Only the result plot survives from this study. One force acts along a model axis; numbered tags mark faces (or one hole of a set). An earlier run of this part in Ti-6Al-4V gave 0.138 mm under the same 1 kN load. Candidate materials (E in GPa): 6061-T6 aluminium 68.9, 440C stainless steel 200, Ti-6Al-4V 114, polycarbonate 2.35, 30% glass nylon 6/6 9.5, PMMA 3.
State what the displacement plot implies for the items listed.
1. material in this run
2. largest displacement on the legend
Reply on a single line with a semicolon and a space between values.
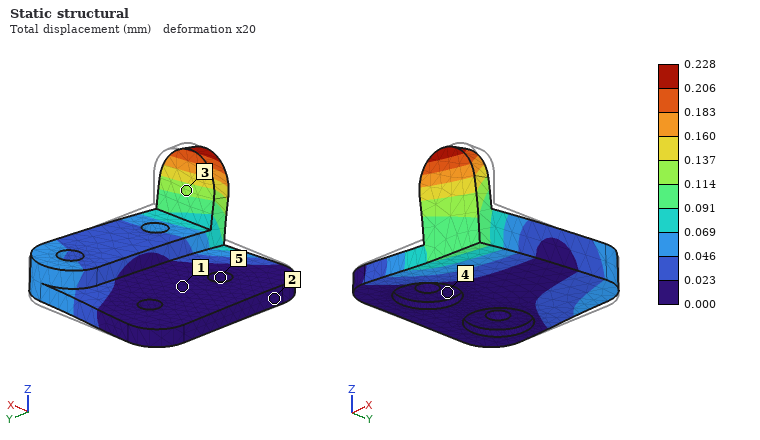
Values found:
6061-T6 aluminium; 0.228 mm
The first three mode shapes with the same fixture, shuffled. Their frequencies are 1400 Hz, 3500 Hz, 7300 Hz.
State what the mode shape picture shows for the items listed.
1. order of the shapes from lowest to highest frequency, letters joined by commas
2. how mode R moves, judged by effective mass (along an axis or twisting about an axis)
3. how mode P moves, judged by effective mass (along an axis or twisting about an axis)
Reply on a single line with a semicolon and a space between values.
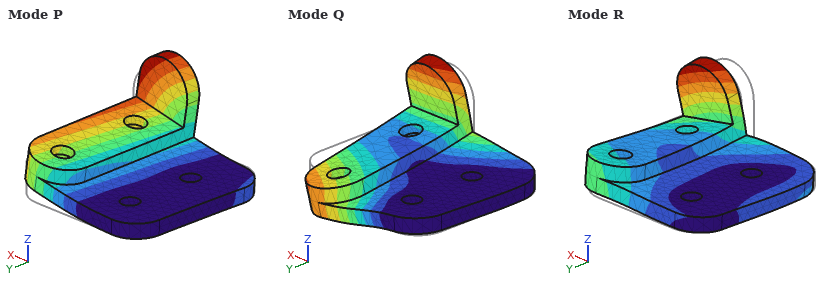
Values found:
P, Q, R; along Y; along Z
